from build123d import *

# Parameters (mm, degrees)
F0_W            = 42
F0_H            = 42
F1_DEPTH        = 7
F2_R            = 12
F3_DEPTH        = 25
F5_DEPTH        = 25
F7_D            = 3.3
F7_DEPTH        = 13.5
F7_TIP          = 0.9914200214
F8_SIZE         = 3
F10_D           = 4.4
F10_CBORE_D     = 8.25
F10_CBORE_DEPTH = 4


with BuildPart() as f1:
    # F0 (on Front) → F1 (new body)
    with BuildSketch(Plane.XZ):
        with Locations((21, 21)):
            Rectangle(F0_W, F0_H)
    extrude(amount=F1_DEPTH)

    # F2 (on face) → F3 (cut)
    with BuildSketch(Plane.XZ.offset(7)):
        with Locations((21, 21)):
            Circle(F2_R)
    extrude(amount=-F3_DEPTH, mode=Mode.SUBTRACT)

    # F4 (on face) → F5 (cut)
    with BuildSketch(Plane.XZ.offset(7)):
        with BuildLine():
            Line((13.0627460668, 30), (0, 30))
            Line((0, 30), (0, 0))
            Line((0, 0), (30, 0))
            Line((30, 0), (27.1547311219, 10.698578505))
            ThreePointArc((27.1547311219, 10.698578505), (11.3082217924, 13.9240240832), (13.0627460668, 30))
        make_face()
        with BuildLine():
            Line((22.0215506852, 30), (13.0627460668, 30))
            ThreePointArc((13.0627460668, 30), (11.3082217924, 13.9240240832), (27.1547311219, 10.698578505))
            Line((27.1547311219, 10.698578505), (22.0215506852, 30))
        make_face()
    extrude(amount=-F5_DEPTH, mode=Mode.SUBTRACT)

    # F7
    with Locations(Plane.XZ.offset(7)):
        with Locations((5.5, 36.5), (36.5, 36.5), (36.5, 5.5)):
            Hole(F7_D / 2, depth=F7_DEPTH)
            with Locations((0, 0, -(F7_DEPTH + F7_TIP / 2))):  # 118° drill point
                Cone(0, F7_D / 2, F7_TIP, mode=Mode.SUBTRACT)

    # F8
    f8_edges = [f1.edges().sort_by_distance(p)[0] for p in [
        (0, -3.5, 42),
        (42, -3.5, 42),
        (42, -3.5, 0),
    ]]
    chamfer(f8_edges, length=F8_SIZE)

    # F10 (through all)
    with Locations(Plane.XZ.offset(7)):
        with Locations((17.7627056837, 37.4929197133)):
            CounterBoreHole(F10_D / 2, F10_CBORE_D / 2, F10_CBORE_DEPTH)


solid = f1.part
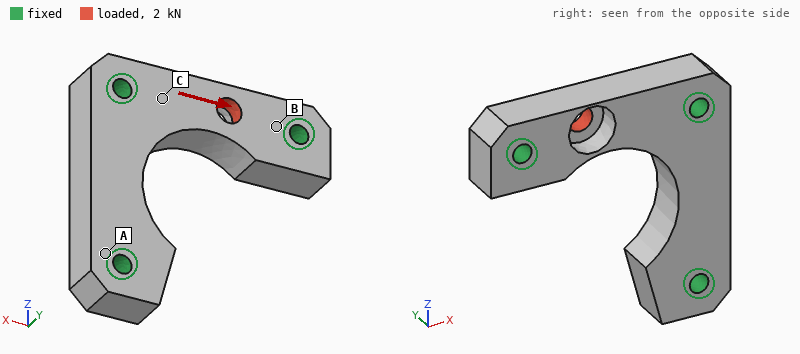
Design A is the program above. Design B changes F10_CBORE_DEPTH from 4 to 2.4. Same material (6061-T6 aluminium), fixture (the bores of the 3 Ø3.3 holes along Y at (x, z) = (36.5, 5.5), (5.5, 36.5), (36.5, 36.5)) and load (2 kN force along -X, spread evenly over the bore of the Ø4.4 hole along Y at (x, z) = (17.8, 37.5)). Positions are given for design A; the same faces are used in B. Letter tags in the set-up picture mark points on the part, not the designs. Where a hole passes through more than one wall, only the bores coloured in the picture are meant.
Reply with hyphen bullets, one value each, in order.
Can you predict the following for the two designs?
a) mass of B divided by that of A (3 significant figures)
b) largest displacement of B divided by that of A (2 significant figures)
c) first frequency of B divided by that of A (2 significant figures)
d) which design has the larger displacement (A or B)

- 1.01
- 0.78
- 1.0
- A
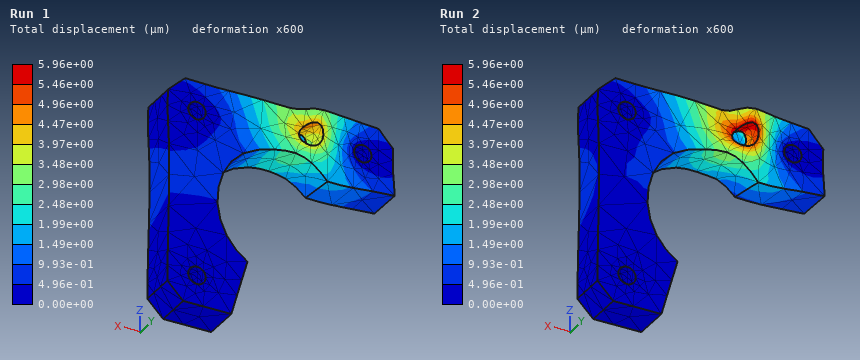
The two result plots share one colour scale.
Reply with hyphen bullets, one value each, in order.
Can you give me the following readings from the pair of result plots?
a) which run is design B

- Run 1
